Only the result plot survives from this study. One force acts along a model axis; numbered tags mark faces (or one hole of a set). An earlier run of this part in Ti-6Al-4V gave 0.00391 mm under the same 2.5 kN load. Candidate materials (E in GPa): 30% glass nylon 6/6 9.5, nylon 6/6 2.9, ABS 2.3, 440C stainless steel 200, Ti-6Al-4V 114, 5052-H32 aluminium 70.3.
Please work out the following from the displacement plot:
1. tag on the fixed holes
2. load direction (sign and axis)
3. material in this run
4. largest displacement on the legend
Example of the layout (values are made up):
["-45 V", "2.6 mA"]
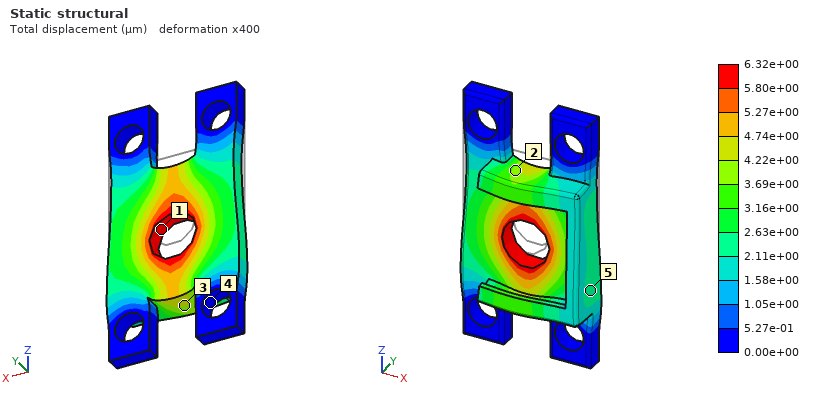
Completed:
["4", "-Z", "5052-H32 aluminium", "6.32e+00 µm"]
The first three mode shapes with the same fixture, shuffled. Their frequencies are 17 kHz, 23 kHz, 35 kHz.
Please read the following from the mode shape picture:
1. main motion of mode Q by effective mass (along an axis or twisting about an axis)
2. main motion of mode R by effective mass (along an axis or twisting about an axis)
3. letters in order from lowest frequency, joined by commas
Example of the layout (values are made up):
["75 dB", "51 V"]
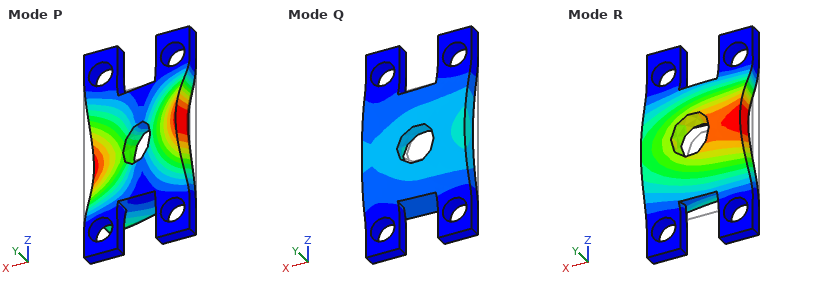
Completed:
["along X", "along Y", "R, P, Q"]
